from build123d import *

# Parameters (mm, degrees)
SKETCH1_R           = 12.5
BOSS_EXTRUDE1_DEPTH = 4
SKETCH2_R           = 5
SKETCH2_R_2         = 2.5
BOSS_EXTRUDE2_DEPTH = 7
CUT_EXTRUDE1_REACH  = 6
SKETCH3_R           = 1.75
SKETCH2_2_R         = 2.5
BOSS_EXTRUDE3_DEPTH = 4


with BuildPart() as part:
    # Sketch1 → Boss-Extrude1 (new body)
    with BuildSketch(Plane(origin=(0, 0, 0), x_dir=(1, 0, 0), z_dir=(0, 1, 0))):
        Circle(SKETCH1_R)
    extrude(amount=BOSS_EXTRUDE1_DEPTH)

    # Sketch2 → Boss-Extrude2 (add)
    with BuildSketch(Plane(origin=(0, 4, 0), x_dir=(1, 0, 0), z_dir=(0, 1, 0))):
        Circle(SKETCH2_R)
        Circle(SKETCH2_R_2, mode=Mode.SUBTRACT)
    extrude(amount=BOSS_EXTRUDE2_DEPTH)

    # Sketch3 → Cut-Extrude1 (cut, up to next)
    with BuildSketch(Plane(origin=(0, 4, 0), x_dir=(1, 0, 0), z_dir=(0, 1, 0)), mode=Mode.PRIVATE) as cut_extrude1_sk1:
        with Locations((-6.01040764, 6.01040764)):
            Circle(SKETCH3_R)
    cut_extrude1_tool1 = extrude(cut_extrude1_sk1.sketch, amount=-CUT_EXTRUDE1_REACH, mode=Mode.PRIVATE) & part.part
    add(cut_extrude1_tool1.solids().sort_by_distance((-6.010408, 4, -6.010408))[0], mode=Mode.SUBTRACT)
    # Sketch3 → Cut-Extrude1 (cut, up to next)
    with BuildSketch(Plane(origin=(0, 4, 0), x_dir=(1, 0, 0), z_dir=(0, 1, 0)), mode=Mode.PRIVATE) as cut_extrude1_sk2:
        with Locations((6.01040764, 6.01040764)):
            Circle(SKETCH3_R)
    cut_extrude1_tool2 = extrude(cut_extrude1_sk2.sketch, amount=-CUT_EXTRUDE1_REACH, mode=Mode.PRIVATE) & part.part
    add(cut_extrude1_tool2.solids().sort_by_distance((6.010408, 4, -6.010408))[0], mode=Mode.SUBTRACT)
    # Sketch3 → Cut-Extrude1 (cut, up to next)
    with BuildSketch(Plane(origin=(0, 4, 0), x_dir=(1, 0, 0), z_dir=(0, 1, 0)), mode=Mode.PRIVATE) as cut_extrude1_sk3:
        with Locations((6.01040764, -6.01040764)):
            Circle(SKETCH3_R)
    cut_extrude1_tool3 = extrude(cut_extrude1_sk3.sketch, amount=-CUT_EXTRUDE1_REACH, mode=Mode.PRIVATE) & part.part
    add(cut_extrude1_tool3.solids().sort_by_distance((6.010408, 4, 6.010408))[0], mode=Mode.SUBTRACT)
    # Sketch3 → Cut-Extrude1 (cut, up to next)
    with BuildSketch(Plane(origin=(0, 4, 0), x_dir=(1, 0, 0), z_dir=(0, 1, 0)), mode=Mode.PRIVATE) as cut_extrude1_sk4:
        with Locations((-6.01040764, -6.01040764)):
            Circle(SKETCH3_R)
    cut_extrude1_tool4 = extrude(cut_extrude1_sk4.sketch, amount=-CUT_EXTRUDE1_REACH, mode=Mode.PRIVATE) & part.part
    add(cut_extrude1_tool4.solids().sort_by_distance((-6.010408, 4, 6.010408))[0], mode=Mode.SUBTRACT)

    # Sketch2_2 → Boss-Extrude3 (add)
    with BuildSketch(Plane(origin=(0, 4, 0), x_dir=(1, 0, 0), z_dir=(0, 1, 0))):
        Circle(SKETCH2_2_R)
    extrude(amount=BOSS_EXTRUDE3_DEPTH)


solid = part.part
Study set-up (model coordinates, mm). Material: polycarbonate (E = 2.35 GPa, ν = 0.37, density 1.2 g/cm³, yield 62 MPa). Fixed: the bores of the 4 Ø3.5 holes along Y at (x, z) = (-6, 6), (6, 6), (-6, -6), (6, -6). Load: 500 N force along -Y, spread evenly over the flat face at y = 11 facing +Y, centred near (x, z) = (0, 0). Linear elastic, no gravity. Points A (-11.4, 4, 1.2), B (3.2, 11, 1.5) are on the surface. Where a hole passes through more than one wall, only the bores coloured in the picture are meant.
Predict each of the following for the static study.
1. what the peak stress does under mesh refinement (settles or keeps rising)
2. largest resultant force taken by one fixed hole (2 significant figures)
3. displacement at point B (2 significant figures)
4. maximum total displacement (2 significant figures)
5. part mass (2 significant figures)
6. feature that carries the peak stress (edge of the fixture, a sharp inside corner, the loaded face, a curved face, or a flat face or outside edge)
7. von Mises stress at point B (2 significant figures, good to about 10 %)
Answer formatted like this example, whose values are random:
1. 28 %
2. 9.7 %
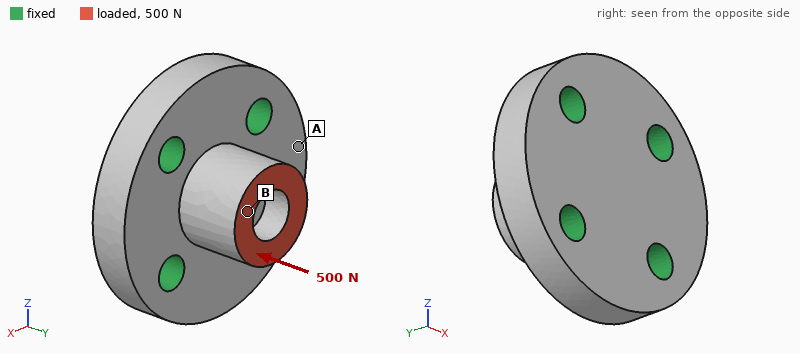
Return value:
1. keeps rising
2. 130 N
3. 48 µm
4. 49 µm
5. 2.8 g
6. edge of the fixture
7. 9.1 MPa
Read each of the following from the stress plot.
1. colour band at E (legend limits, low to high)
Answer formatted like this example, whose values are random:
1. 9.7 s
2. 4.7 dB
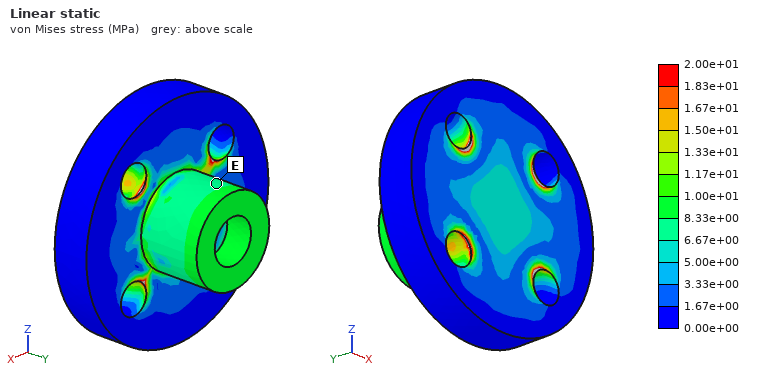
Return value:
1. 6.67e+00 to 8.33e+00 MPa
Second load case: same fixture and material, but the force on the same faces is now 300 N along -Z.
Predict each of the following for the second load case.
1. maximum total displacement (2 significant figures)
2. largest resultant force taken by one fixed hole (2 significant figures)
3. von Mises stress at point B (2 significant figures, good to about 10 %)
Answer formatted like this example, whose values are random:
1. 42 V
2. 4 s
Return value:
1. 0.17 mm
2. 150 N
3. 12 MPa
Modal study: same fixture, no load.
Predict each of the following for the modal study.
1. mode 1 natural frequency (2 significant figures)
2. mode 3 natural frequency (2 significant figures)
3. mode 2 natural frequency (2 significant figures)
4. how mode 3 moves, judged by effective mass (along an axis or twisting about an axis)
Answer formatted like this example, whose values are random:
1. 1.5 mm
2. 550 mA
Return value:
1. 16 kHz
2. 20 kHz
3. 16 kHz
4. along Y
